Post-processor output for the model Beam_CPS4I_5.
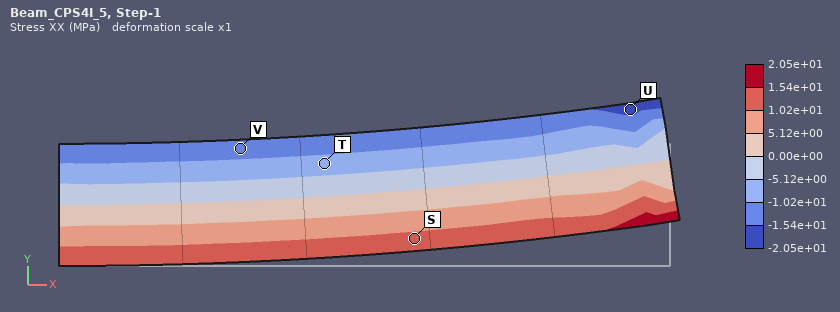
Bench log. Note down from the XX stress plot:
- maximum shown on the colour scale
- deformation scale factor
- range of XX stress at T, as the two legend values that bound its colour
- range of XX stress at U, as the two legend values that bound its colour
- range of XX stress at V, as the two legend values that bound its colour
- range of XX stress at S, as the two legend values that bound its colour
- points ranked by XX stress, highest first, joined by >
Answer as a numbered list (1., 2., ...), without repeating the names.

1. 2.05e+01 MPa
2. 1
3. -1.02e+01 to -5.12e+00 MPa
4. -2.05e+01 to -1.54e+01 MPa
5. -1.54e+01 to -1.02e+01 MPa
6. 1.02e+01 to 1.54e+01 MPa
7. S > T > V > U
